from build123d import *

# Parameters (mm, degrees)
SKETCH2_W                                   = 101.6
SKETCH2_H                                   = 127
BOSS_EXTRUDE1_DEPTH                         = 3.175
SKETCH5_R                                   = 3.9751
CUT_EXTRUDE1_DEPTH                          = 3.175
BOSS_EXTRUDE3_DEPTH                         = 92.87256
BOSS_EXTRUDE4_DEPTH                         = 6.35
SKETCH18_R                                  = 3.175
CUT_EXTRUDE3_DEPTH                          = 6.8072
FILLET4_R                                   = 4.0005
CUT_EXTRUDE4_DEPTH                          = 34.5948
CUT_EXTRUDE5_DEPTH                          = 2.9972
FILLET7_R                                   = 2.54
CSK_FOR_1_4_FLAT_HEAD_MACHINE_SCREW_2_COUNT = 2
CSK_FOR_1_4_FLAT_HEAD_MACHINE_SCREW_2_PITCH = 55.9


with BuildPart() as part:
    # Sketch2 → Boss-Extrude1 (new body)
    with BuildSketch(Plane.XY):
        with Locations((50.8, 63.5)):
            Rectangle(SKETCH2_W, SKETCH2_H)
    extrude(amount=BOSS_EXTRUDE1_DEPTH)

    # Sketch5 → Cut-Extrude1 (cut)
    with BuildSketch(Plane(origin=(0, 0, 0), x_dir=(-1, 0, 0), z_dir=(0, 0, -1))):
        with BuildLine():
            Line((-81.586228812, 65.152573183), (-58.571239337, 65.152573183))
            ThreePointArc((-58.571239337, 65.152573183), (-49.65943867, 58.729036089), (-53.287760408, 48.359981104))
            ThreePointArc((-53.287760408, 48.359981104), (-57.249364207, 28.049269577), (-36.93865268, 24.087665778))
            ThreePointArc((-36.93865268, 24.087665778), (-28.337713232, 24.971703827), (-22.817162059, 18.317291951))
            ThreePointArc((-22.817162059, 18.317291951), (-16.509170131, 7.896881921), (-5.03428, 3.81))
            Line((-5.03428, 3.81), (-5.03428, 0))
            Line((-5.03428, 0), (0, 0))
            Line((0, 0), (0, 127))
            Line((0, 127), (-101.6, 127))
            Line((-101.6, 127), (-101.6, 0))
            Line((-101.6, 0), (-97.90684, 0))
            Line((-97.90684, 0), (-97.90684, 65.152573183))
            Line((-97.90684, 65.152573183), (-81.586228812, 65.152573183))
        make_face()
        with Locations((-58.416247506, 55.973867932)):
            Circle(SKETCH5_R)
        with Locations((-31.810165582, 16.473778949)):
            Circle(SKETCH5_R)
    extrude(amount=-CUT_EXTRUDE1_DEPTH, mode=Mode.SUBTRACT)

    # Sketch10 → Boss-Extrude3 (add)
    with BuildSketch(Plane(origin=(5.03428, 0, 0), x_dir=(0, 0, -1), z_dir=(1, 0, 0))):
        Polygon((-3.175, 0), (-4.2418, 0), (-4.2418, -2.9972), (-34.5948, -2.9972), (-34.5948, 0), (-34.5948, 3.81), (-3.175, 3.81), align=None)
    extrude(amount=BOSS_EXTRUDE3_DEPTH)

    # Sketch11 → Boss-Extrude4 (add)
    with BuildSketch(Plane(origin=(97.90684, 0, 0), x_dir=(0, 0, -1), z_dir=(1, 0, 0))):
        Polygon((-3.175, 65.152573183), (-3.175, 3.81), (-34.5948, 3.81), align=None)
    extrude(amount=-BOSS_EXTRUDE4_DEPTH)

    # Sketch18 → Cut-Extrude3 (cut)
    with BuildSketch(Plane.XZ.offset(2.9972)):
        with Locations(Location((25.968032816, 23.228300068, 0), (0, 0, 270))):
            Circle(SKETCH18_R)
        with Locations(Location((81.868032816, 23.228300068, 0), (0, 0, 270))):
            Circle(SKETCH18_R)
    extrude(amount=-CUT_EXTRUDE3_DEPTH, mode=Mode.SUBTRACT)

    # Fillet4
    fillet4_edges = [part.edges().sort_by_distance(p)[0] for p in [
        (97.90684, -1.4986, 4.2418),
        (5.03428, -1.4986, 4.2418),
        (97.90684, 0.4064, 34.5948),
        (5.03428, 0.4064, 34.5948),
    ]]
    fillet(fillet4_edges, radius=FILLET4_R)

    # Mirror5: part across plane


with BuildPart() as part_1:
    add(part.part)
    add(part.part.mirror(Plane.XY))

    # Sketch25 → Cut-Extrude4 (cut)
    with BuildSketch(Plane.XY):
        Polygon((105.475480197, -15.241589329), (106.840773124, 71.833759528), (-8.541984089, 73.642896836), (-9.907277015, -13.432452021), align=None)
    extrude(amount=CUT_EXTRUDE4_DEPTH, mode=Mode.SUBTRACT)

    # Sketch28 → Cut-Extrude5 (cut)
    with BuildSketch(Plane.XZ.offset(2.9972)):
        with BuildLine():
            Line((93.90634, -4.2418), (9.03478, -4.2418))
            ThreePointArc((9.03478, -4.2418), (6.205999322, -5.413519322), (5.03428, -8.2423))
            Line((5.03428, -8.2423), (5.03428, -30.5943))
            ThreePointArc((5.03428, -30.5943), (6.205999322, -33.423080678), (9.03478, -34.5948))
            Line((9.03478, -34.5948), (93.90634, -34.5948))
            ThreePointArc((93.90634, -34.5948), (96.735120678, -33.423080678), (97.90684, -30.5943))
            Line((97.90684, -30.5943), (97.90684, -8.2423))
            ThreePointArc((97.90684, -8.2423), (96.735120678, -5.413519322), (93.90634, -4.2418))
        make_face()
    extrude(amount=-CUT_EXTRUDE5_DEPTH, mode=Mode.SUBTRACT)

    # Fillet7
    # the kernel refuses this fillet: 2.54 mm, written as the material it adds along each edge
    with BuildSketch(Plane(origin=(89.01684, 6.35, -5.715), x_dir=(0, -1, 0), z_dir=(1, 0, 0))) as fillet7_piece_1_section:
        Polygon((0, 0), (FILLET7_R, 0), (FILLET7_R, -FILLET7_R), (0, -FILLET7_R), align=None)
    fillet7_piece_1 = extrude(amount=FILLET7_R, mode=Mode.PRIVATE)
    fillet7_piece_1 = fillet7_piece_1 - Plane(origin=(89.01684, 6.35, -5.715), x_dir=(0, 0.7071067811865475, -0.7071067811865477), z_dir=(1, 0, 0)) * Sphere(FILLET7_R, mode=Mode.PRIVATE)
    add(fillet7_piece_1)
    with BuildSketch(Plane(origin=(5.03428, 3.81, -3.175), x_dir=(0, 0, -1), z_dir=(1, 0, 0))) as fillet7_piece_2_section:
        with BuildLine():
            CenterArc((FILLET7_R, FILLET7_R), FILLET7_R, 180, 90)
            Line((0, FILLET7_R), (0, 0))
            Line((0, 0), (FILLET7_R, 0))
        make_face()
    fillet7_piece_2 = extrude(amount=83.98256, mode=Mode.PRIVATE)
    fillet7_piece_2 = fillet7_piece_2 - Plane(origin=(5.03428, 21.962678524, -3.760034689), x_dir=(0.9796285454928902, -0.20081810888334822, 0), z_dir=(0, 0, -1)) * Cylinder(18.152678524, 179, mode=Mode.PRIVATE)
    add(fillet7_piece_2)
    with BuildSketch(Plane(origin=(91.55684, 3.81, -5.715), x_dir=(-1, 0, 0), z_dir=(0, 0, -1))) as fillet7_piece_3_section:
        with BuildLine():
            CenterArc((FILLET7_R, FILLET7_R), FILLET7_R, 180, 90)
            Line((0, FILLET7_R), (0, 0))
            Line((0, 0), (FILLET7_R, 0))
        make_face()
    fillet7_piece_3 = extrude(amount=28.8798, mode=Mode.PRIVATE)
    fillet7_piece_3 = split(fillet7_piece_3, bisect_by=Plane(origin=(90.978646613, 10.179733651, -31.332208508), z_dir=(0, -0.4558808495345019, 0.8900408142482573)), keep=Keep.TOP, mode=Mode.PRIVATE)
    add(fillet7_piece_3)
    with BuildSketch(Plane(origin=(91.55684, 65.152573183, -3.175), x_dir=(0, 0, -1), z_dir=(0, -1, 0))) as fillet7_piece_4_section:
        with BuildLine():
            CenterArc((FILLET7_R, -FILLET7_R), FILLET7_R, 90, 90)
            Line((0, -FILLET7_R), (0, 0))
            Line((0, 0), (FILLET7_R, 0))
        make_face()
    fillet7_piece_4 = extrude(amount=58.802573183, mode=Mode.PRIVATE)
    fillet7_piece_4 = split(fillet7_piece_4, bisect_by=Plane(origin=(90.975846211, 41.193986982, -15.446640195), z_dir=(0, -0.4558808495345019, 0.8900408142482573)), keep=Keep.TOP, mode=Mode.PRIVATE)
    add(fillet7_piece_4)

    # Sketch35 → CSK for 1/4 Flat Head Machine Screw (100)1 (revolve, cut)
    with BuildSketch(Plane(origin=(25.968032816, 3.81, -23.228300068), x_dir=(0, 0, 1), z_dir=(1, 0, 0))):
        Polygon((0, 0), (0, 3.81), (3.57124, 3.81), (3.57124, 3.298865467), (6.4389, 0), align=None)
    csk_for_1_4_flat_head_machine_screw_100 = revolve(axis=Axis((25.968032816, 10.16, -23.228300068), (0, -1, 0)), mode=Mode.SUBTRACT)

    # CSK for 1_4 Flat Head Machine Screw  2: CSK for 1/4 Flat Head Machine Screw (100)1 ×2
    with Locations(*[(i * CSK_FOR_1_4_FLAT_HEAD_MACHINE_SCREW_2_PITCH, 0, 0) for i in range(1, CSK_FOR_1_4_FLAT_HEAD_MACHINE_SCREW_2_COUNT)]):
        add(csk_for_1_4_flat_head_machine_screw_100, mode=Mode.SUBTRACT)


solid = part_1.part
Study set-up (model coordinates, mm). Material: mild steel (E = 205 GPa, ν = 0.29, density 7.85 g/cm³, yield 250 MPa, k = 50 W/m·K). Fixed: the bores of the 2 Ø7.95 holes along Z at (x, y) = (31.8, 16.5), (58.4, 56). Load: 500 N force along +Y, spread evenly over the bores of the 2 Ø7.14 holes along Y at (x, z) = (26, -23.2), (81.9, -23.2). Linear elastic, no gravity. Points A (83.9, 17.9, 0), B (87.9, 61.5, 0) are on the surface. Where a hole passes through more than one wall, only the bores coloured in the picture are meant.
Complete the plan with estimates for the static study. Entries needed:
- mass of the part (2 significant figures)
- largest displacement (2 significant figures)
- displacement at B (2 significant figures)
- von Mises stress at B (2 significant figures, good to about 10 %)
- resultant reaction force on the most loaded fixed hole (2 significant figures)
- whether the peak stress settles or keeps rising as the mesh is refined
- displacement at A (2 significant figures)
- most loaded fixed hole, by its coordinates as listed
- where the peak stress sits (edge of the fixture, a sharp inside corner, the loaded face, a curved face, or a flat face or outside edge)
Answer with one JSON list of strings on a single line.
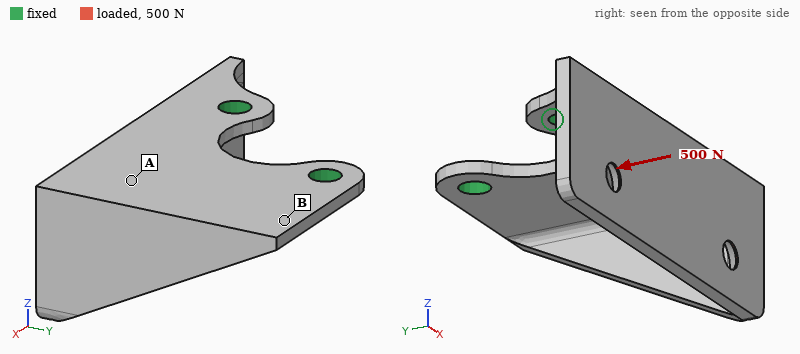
["220 g", "0.13 mm", "0.023 mm", "32 MPa", "350 N", "keeps rising", "0.047 mm", "(31.8, 16.5)", "edge of the fixture"]
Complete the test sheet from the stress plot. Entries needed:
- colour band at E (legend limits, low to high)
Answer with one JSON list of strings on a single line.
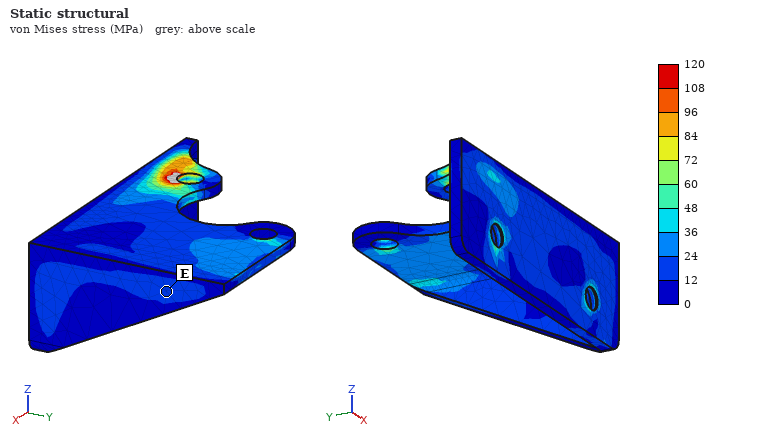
["12 to 24 MPa"]
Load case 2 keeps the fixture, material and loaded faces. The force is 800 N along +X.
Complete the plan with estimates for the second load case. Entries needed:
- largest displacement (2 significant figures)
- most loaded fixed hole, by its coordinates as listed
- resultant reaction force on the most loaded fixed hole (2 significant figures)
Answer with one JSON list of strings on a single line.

["0.28 mm", "(31.8, 16.5)", "850 N"]
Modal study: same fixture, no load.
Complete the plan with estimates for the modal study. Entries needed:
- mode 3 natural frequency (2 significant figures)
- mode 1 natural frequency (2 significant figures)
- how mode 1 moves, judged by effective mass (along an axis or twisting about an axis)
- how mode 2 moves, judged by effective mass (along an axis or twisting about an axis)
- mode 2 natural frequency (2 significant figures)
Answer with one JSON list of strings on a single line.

["2200 Hz", "610 Hz", "along Z", "along Y", "1500 Hz"]
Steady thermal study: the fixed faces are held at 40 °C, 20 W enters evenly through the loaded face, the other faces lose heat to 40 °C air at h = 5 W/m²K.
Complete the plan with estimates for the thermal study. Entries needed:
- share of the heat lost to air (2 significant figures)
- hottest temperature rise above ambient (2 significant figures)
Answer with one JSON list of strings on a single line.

["15 %", "80 K"]
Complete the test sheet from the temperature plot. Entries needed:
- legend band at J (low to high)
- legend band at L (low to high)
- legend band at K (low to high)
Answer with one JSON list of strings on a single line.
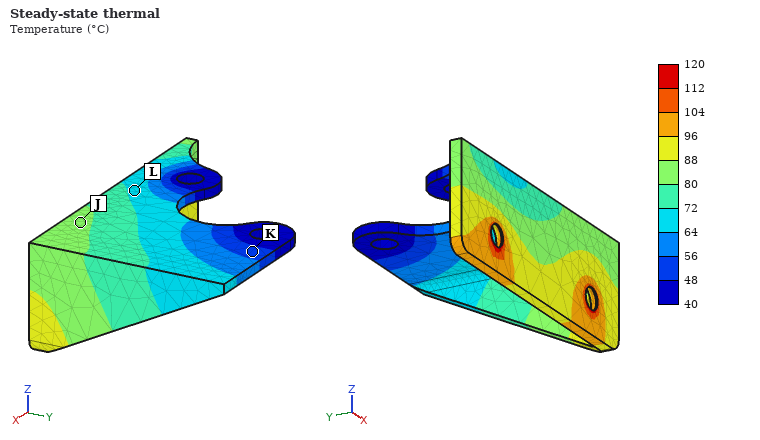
["80 to 88 °C", "64 to 72 °C", "48 to 56 °C"]
